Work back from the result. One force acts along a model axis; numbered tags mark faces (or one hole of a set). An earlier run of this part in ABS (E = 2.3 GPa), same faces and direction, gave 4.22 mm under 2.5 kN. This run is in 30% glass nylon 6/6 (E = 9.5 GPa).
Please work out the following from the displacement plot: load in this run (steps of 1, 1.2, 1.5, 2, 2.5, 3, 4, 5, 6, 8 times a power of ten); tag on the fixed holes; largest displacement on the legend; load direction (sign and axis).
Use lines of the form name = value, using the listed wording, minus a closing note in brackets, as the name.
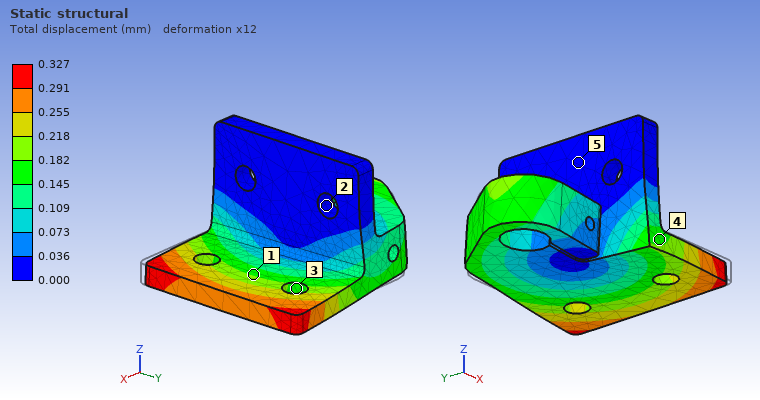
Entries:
load in this run = 800 N
tag on the fixed holes = 2
largest displacement on the legend = 0.327 mm
load direction = +Y
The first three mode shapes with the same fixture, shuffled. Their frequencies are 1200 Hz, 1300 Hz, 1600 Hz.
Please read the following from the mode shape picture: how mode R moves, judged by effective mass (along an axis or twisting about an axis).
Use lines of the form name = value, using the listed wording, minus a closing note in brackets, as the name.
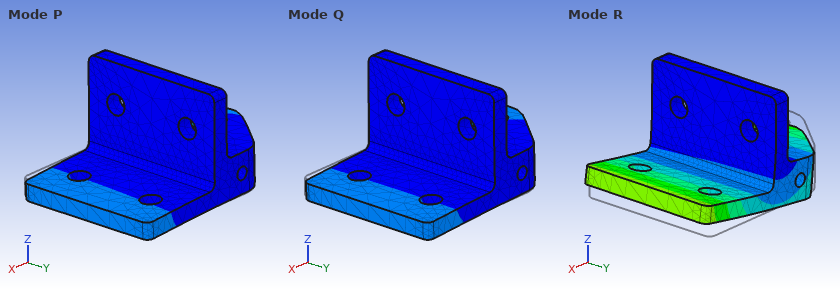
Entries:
how mode R moves, judged by effective mass = along X
